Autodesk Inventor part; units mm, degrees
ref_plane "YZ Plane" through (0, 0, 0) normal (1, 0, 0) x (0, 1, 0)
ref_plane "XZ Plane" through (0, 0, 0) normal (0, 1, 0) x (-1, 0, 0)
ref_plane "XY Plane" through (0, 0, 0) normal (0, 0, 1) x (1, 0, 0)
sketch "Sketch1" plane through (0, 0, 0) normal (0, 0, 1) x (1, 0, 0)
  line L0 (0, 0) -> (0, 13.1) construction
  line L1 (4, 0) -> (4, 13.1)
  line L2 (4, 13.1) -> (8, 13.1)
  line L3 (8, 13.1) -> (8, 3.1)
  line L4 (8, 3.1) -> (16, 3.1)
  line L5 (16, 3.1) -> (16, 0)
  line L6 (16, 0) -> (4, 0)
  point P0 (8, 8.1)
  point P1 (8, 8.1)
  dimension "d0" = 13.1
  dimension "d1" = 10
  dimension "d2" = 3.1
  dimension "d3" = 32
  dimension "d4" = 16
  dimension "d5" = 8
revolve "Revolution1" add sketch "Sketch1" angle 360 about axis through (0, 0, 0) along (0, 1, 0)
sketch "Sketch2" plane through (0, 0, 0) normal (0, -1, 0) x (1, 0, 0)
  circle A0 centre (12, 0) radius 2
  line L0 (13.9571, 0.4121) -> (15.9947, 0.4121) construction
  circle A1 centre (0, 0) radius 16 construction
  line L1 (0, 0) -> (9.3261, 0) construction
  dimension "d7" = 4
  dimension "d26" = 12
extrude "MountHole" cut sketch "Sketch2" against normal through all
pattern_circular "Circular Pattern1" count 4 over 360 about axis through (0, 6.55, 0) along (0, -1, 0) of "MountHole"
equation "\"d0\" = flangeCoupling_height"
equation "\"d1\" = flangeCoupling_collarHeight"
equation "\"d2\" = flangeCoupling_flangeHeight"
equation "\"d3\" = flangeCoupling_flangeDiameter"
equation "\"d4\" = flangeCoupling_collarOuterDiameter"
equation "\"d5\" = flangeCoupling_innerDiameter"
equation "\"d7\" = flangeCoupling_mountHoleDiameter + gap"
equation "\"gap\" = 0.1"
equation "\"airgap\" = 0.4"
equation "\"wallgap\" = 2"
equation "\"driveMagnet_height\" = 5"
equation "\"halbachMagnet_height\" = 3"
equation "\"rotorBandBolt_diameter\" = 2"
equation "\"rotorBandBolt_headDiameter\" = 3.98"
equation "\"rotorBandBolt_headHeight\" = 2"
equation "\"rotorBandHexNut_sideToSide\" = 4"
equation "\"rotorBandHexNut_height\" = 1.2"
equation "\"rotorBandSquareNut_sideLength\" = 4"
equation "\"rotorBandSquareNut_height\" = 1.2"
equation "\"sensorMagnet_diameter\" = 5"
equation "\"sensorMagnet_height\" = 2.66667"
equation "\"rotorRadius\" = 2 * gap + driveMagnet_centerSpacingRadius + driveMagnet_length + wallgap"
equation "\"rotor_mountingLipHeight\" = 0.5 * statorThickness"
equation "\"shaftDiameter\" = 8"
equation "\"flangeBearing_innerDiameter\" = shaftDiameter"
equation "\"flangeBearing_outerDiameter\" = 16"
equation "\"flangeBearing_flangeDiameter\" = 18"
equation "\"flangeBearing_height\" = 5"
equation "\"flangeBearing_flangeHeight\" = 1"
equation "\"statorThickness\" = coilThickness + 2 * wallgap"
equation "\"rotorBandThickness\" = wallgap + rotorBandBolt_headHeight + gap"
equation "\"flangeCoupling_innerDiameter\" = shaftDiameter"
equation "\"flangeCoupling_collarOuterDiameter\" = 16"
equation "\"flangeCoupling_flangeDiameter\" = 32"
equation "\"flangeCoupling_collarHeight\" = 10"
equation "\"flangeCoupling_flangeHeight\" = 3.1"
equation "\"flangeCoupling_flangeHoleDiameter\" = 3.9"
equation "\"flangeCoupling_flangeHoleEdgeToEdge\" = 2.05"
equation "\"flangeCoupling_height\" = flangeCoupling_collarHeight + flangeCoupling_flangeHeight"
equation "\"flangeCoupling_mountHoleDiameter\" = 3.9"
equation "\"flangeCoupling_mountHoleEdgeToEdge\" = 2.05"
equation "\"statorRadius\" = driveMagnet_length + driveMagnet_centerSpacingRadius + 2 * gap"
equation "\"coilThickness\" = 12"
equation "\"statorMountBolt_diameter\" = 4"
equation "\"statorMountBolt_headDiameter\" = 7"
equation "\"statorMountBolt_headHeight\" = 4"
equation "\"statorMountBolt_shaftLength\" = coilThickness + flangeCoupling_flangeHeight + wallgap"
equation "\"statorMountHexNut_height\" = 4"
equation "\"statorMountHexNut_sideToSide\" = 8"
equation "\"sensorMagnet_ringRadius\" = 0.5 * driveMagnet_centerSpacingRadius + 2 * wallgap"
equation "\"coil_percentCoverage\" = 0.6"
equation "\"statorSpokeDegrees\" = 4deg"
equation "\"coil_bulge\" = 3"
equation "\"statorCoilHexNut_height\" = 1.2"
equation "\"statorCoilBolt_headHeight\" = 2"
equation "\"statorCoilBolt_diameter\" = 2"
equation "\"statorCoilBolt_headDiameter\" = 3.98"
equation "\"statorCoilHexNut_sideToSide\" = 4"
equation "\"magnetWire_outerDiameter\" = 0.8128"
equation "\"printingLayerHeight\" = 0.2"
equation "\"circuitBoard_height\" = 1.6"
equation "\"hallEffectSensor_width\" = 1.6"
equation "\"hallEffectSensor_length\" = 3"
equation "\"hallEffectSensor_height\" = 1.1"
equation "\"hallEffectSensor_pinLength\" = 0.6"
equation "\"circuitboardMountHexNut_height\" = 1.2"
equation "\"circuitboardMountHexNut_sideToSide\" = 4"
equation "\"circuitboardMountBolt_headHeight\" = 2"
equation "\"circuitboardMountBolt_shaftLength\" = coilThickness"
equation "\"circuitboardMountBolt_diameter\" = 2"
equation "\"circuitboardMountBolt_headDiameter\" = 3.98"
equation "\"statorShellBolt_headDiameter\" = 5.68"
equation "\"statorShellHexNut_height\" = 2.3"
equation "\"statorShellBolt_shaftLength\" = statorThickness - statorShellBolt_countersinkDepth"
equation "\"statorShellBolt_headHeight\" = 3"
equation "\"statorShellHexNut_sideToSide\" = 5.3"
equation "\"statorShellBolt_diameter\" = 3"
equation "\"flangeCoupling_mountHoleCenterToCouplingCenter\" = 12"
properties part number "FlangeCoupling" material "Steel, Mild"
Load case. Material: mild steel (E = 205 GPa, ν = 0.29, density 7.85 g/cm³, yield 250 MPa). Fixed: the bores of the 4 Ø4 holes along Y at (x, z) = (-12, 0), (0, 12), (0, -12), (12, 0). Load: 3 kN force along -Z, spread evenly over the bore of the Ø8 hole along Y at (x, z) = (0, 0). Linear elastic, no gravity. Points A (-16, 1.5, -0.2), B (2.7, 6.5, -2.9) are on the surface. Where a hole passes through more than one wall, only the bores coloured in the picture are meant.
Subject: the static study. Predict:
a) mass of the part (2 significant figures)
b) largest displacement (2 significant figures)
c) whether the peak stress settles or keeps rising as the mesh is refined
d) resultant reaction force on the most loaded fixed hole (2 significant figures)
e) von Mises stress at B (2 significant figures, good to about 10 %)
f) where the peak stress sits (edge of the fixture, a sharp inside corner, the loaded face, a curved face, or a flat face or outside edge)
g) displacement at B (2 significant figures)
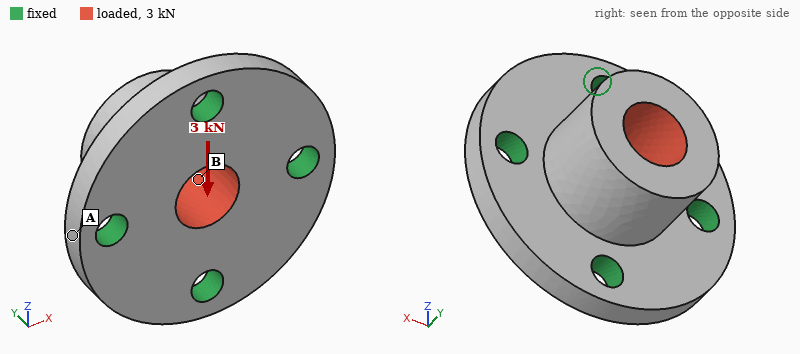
29 g
6.1 µm
keeps rising
1.2 kN
30 MPa
edge of the fixture
2.8 µm
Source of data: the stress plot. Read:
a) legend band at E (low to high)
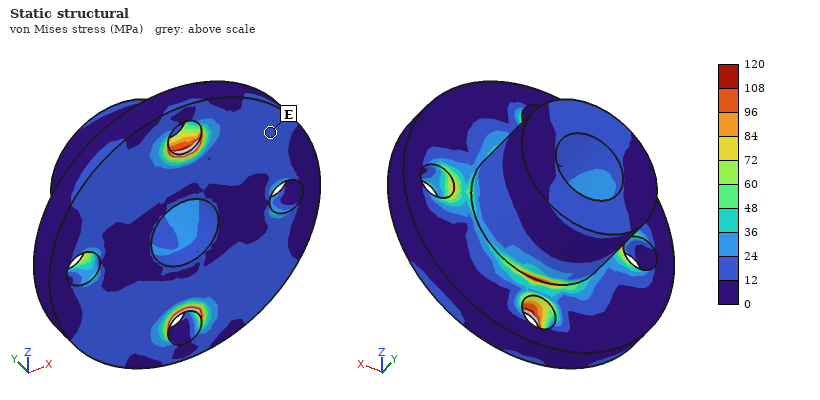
12 to 24 MPa
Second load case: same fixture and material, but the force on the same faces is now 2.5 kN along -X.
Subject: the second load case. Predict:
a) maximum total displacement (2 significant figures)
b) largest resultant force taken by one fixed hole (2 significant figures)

5.0 µm
1.0 kN
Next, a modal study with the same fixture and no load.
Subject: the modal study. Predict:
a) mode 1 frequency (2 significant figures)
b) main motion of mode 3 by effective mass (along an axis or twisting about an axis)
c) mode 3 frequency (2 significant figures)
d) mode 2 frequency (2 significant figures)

32 kHz
along Y
39 kHz
32 kHz
